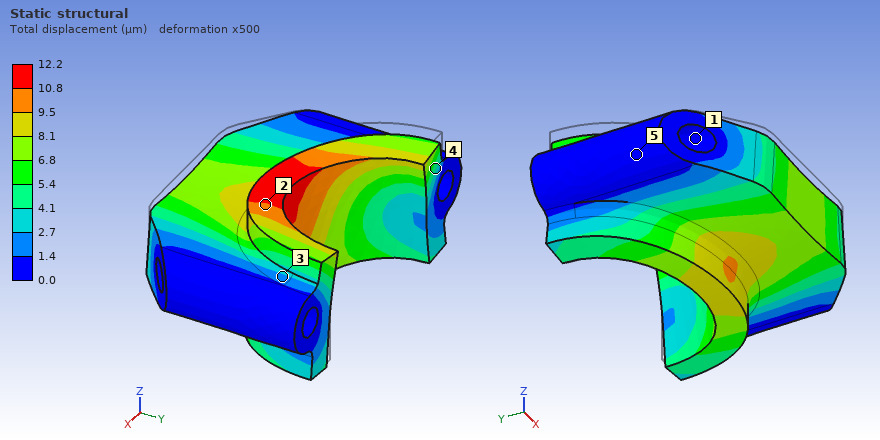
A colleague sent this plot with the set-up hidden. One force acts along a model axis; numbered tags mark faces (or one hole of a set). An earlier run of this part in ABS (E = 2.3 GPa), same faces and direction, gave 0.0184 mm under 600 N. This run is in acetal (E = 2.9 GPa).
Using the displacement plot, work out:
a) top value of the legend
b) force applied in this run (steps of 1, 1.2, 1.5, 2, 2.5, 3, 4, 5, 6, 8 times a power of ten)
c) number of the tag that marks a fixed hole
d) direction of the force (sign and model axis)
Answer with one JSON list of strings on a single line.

["12.2 µm", "500 N", "1", "-Z"]
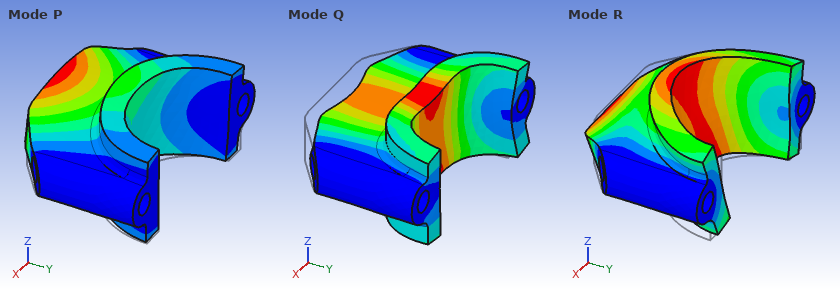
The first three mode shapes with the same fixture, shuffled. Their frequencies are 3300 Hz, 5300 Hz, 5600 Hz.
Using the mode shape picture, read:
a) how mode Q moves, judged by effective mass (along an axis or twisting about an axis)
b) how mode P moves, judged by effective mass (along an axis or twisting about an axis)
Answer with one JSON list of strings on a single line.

["along Y", "along Z"]
